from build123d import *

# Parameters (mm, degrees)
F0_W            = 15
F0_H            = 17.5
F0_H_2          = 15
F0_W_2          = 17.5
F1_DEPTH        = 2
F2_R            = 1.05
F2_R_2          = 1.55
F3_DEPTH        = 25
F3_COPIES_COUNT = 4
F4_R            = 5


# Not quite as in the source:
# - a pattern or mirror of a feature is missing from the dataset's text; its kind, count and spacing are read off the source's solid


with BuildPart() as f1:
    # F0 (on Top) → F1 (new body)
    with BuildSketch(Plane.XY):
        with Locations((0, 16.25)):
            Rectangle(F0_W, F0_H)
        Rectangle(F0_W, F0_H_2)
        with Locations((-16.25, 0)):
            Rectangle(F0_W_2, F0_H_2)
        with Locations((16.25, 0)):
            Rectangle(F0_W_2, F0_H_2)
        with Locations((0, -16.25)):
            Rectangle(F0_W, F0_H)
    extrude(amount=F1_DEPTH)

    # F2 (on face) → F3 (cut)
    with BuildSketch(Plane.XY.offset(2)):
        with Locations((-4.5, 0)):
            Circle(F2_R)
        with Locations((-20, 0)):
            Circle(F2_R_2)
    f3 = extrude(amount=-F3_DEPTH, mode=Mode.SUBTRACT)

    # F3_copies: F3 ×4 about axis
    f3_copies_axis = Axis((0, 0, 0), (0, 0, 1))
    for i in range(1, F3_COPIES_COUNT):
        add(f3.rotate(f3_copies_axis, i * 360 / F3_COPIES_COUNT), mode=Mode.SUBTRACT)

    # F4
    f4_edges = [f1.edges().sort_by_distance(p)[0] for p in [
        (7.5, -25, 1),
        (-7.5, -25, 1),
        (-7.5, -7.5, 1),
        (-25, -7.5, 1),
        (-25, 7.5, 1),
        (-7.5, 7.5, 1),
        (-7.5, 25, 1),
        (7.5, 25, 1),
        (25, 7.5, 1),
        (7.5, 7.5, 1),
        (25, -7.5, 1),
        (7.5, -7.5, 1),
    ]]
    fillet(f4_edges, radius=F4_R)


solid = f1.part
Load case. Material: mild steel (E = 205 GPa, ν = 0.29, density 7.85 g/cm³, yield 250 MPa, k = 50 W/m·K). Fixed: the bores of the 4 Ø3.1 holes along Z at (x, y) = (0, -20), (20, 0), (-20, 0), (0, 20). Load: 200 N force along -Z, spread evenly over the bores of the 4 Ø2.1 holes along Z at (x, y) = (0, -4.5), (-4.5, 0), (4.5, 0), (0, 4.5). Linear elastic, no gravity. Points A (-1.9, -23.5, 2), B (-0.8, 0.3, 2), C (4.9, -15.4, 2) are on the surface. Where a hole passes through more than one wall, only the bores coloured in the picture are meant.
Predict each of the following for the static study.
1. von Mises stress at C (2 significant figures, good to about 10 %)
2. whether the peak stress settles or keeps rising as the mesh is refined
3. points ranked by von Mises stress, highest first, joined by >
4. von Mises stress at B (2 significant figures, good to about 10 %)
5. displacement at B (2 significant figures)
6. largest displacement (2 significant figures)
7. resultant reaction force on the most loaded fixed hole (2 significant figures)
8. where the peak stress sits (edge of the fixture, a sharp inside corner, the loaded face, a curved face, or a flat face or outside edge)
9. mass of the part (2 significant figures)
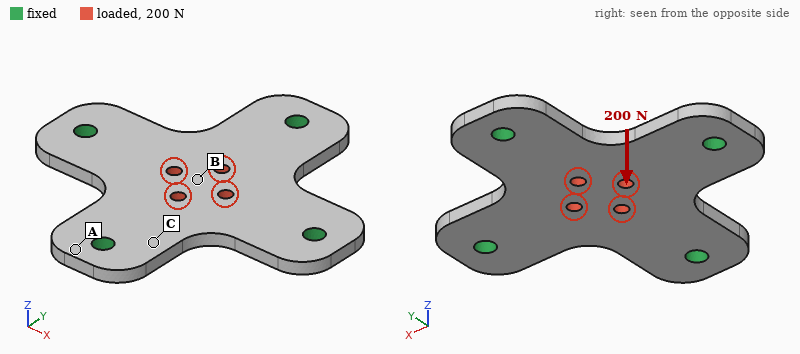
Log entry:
19 MPa
keeps rising
B > C > A
36 MPa
13 µm
13 µm
50 N
edge of the fixture
19 g
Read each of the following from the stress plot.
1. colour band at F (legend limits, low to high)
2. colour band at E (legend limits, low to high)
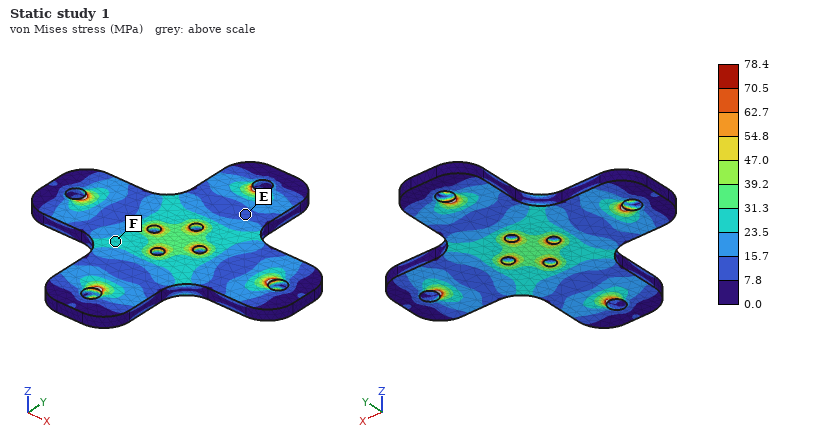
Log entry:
23.5 to 31.3 MPa
7.8 to 15.7 MPa
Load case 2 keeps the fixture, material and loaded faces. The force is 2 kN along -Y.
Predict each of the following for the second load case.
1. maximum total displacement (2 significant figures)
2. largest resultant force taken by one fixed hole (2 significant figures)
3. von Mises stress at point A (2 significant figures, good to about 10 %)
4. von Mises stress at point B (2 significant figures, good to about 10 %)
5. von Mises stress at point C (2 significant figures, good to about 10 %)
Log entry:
3.6 µm
850 N
19 MPa
8.7 MPa
24 MPa
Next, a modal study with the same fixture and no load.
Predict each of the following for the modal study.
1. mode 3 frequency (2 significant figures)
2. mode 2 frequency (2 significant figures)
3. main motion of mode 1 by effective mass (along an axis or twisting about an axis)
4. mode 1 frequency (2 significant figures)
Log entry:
18 kHz
18 kHz
along Z
9600 Hz
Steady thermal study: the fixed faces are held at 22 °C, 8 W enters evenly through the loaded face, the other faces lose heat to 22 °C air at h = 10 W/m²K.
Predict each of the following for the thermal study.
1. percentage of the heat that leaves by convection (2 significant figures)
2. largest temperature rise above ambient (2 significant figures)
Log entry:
3.3 %
28 K
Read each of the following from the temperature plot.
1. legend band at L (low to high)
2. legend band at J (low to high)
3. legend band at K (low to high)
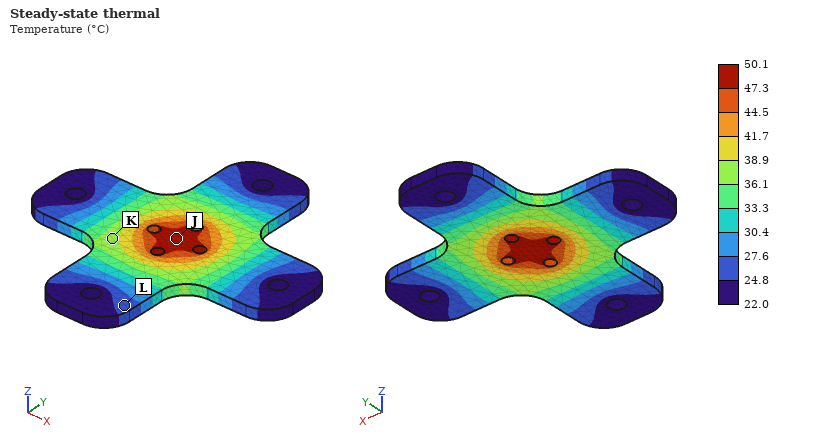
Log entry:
24.8 to 27.6 °C
47.3 to 50.1 °C
36.1 to 38.9 °C
